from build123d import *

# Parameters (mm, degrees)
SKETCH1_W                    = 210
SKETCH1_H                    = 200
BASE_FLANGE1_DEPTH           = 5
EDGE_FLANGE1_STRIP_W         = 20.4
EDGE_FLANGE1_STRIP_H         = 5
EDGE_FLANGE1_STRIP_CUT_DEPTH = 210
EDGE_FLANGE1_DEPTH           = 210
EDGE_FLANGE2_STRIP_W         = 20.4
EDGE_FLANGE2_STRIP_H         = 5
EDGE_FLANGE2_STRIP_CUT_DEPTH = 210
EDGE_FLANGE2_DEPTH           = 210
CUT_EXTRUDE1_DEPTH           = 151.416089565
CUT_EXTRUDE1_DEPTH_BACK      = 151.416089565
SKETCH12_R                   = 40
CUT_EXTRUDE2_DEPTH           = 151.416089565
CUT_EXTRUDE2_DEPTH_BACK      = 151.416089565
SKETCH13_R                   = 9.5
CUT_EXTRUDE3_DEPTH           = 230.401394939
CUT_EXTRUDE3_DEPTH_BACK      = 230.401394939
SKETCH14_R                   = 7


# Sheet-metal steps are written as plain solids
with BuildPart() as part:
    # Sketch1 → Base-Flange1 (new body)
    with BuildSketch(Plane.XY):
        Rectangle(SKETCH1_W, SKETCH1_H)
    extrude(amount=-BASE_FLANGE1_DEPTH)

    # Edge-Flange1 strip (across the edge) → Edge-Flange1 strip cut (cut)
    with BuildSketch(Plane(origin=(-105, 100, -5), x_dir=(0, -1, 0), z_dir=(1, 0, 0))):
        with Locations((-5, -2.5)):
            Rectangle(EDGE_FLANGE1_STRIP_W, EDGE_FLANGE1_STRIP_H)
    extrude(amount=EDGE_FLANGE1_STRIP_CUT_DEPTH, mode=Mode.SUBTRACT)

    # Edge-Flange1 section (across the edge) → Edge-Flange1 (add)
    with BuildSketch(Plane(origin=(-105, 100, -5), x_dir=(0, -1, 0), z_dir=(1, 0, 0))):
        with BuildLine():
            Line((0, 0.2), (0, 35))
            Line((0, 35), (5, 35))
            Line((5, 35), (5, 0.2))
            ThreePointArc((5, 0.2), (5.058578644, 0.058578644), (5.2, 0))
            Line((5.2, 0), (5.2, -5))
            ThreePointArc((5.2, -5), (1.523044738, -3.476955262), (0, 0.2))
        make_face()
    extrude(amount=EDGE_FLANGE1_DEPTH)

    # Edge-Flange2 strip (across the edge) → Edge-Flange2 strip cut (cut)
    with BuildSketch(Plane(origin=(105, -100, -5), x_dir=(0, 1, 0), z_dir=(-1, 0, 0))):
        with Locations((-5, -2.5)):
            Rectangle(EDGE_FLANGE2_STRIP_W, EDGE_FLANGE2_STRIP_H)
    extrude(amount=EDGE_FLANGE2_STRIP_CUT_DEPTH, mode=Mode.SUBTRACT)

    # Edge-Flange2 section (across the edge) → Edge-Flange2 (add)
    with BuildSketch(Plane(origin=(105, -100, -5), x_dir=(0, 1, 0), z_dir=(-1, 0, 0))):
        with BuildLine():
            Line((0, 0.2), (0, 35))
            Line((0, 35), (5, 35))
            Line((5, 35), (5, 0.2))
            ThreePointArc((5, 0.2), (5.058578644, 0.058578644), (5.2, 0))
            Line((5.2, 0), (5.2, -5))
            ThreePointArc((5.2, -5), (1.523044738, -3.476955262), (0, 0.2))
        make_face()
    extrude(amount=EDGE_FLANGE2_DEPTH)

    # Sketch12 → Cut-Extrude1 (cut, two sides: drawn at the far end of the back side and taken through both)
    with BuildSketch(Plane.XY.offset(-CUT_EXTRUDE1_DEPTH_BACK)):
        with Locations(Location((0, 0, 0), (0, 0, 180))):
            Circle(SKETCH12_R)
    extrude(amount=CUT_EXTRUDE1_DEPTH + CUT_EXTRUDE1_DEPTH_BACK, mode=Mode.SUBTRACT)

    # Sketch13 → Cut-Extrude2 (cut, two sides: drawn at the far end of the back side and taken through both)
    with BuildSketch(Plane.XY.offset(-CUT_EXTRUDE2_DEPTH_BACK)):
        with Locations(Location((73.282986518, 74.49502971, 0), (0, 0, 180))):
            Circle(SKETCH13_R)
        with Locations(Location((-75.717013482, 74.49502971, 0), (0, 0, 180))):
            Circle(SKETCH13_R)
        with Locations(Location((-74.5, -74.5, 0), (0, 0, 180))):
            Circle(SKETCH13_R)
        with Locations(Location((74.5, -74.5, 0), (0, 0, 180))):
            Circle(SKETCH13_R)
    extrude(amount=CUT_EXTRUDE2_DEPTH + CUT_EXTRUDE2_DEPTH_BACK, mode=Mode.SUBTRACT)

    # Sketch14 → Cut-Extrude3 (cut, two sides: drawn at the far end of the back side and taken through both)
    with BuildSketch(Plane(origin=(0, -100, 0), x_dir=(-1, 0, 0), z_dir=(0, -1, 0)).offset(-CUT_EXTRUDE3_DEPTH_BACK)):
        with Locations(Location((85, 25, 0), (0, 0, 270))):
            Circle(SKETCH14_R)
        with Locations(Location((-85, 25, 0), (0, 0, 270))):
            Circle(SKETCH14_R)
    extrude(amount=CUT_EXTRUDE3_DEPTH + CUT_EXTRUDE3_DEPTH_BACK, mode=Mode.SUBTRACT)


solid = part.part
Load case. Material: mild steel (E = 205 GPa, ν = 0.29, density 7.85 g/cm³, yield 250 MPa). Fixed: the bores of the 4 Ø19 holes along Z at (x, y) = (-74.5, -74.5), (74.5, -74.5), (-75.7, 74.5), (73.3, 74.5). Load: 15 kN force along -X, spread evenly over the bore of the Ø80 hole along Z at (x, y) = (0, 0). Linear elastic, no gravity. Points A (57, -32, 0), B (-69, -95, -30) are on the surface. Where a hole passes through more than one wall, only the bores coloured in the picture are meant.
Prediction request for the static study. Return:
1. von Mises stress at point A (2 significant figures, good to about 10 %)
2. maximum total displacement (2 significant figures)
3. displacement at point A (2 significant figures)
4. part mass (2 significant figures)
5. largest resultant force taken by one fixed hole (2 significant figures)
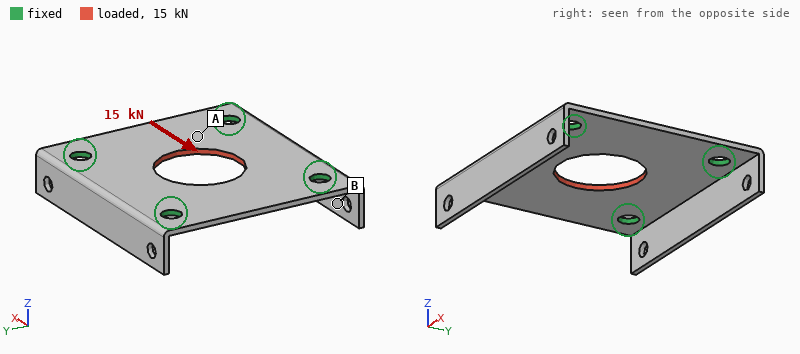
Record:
13 MPa
7.7 µm
4.8 µm
1.9 kg
4.0 kN
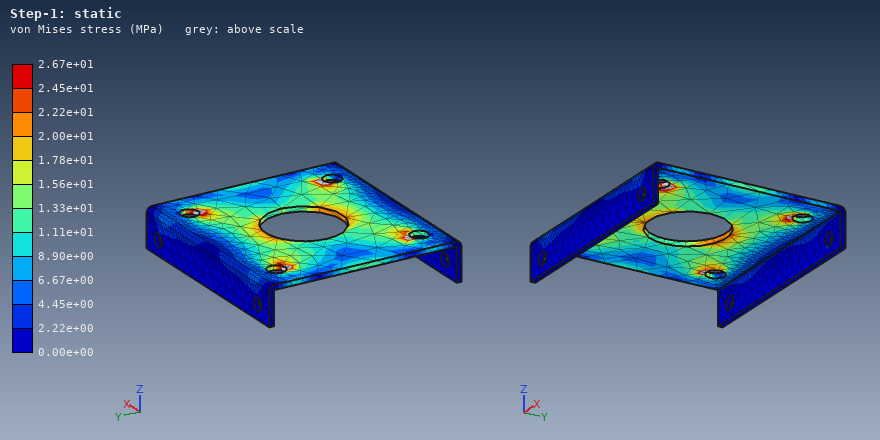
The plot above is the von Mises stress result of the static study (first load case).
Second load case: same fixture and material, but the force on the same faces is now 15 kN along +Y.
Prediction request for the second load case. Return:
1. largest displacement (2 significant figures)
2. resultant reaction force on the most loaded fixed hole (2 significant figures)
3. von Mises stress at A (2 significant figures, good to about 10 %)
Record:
7.8 µm
4.0 kN
13 MPa
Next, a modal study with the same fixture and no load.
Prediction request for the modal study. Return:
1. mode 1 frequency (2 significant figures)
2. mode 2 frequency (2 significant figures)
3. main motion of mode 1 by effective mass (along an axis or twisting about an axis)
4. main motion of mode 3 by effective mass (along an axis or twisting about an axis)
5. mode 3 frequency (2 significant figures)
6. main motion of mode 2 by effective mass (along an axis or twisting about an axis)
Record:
1200 Hz
1400 Hz
along Z
along Y
1500 Hz
twisting about Y
